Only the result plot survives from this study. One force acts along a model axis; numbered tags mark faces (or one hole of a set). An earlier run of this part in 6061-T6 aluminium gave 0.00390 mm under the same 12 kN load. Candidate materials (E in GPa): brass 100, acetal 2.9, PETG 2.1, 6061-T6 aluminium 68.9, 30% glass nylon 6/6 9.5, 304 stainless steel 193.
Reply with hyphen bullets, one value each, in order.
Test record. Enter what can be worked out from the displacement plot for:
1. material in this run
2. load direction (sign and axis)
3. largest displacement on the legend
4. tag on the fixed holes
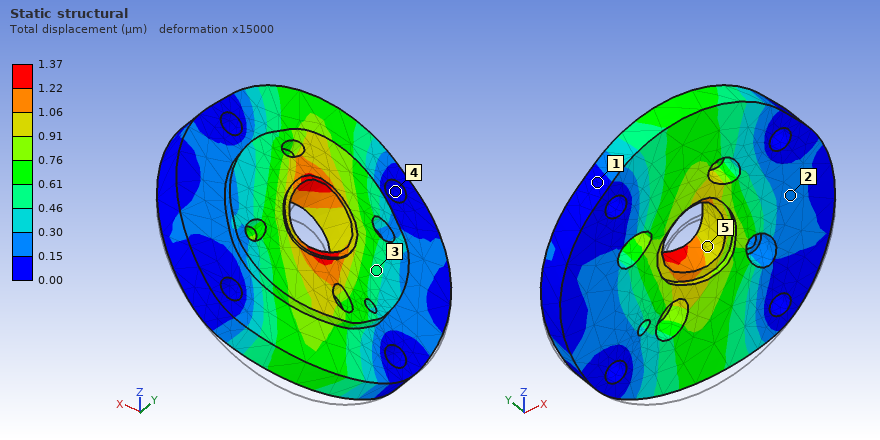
- 304 stainless steel
- +Z
- 1.37 µm
- 4
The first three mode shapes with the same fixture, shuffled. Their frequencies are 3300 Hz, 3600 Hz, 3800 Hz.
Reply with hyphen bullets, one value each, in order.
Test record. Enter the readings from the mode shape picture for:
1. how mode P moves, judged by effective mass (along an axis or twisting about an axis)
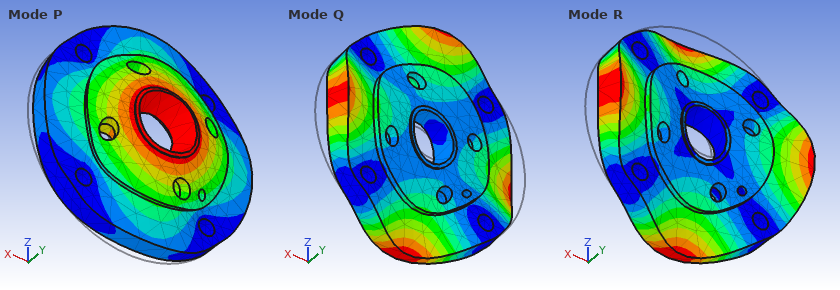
- along Y
